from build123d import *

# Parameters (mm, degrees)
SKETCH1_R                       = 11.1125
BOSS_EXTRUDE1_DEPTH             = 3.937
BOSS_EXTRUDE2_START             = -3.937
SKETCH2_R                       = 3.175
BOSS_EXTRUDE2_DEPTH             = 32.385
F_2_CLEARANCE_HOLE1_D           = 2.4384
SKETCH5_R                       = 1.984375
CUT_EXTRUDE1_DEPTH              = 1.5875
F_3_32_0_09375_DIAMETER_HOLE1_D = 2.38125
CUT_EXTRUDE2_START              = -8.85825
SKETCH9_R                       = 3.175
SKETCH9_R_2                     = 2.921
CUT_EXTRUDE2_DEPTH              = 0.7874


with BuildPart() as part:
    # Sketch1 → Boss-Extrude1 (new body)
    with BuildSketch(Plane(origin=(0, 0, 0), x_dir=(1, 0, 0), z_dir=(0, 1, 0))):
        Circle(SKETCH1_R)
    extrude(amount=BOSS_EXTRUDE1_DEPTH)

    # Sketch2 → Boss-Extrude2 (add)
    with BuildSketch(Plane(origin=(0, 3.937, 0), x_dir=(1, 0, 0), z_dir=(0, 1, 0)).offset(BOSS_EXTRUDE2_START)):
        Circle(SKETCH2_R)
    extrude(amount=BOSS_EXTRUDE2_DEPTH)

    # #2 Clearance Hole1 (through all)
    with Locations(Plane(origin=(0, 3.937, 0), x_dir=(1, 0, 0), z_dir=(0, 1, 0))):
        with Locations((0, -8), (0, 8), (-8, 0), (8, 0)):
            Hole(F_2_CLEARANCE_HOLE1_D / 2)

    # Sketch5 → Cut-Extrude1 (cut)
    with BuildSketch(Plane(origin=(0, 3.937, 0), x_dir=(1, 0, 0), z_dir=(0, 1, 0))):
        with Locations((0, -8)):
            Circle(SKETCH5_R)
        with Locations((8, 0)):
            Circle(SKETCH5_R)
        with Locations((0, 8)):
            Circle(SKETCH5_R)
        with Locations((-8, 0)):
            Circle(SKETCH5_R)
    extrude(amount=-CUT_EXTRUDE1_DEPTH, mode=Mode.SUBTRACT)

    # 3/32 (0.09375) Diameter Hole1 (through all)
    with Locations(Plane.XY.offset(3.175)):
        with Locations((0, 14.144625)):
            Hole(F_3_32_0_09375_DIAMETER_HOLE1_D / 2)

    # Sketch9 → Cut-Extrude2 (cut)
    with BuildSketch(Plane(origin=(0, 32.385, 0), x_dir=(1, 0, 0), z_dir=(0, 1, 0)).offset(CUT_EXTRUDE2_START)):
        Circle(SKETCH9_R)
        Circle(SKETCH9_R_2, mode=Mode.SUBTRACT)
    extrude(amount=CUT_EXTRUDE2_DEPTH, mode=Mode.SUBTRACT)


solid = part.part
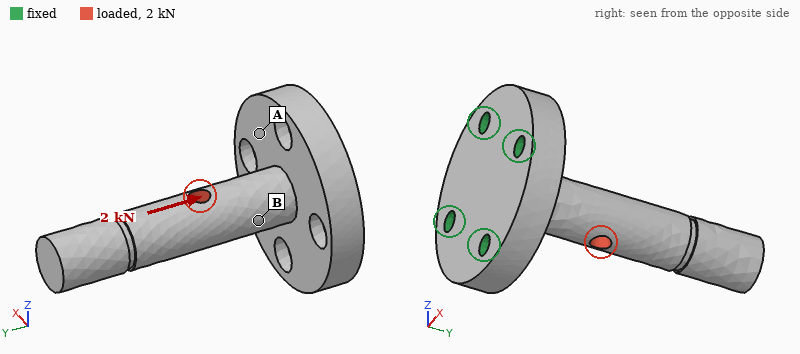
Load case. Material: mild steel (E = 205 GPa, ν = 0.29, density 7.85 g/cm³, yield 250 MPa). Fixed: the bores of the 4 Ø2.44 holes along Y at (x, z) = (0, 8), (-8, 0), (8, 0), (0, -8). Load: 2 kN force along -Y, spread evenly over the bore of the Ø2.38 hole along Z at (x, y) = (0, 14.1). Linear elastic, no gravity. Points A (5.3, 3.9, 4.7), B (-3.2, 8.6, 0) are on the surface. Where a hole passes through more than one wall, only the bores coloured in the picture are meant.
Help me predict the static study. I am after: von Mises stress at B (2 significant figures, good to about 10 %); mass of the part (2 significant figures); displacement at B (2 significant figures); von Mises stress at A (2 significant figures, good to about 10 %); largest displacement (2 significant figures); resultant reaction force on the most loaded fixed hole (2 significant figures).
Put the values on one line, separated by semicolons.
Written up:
64 MPa; 18 g; 4.5 µm; 24 MPa; 7.1 µm; 580 N
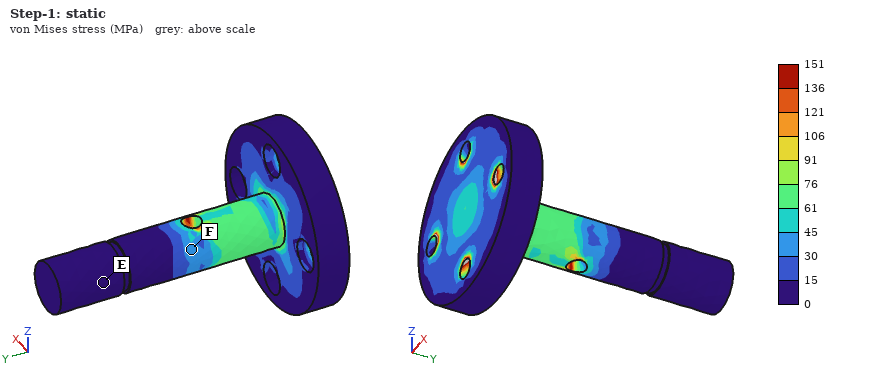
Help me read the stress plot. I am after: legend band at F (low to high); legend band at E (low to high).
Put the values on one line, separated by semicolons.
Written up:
30 to 45 MPa; 0 to 15 MPa
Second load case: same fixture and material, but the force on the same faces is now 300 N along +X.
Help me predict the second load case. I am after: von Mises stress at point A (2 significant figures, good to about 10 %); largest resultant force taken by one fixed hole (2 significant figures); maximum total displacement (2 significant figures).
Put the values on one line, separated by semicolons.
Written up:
9.1 MPa; 290 N; 38 µm
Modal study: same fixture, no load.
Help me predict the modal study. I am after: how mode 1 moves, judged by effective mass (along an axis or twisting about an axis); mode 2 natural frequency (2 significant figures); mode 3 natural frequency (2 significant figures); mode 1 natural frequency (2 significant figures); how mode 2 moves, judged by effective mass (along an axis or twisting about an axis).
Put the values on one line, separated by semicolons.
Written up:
along Z; 4800 Hz; 25 kHz; 4500 Hz; along X
